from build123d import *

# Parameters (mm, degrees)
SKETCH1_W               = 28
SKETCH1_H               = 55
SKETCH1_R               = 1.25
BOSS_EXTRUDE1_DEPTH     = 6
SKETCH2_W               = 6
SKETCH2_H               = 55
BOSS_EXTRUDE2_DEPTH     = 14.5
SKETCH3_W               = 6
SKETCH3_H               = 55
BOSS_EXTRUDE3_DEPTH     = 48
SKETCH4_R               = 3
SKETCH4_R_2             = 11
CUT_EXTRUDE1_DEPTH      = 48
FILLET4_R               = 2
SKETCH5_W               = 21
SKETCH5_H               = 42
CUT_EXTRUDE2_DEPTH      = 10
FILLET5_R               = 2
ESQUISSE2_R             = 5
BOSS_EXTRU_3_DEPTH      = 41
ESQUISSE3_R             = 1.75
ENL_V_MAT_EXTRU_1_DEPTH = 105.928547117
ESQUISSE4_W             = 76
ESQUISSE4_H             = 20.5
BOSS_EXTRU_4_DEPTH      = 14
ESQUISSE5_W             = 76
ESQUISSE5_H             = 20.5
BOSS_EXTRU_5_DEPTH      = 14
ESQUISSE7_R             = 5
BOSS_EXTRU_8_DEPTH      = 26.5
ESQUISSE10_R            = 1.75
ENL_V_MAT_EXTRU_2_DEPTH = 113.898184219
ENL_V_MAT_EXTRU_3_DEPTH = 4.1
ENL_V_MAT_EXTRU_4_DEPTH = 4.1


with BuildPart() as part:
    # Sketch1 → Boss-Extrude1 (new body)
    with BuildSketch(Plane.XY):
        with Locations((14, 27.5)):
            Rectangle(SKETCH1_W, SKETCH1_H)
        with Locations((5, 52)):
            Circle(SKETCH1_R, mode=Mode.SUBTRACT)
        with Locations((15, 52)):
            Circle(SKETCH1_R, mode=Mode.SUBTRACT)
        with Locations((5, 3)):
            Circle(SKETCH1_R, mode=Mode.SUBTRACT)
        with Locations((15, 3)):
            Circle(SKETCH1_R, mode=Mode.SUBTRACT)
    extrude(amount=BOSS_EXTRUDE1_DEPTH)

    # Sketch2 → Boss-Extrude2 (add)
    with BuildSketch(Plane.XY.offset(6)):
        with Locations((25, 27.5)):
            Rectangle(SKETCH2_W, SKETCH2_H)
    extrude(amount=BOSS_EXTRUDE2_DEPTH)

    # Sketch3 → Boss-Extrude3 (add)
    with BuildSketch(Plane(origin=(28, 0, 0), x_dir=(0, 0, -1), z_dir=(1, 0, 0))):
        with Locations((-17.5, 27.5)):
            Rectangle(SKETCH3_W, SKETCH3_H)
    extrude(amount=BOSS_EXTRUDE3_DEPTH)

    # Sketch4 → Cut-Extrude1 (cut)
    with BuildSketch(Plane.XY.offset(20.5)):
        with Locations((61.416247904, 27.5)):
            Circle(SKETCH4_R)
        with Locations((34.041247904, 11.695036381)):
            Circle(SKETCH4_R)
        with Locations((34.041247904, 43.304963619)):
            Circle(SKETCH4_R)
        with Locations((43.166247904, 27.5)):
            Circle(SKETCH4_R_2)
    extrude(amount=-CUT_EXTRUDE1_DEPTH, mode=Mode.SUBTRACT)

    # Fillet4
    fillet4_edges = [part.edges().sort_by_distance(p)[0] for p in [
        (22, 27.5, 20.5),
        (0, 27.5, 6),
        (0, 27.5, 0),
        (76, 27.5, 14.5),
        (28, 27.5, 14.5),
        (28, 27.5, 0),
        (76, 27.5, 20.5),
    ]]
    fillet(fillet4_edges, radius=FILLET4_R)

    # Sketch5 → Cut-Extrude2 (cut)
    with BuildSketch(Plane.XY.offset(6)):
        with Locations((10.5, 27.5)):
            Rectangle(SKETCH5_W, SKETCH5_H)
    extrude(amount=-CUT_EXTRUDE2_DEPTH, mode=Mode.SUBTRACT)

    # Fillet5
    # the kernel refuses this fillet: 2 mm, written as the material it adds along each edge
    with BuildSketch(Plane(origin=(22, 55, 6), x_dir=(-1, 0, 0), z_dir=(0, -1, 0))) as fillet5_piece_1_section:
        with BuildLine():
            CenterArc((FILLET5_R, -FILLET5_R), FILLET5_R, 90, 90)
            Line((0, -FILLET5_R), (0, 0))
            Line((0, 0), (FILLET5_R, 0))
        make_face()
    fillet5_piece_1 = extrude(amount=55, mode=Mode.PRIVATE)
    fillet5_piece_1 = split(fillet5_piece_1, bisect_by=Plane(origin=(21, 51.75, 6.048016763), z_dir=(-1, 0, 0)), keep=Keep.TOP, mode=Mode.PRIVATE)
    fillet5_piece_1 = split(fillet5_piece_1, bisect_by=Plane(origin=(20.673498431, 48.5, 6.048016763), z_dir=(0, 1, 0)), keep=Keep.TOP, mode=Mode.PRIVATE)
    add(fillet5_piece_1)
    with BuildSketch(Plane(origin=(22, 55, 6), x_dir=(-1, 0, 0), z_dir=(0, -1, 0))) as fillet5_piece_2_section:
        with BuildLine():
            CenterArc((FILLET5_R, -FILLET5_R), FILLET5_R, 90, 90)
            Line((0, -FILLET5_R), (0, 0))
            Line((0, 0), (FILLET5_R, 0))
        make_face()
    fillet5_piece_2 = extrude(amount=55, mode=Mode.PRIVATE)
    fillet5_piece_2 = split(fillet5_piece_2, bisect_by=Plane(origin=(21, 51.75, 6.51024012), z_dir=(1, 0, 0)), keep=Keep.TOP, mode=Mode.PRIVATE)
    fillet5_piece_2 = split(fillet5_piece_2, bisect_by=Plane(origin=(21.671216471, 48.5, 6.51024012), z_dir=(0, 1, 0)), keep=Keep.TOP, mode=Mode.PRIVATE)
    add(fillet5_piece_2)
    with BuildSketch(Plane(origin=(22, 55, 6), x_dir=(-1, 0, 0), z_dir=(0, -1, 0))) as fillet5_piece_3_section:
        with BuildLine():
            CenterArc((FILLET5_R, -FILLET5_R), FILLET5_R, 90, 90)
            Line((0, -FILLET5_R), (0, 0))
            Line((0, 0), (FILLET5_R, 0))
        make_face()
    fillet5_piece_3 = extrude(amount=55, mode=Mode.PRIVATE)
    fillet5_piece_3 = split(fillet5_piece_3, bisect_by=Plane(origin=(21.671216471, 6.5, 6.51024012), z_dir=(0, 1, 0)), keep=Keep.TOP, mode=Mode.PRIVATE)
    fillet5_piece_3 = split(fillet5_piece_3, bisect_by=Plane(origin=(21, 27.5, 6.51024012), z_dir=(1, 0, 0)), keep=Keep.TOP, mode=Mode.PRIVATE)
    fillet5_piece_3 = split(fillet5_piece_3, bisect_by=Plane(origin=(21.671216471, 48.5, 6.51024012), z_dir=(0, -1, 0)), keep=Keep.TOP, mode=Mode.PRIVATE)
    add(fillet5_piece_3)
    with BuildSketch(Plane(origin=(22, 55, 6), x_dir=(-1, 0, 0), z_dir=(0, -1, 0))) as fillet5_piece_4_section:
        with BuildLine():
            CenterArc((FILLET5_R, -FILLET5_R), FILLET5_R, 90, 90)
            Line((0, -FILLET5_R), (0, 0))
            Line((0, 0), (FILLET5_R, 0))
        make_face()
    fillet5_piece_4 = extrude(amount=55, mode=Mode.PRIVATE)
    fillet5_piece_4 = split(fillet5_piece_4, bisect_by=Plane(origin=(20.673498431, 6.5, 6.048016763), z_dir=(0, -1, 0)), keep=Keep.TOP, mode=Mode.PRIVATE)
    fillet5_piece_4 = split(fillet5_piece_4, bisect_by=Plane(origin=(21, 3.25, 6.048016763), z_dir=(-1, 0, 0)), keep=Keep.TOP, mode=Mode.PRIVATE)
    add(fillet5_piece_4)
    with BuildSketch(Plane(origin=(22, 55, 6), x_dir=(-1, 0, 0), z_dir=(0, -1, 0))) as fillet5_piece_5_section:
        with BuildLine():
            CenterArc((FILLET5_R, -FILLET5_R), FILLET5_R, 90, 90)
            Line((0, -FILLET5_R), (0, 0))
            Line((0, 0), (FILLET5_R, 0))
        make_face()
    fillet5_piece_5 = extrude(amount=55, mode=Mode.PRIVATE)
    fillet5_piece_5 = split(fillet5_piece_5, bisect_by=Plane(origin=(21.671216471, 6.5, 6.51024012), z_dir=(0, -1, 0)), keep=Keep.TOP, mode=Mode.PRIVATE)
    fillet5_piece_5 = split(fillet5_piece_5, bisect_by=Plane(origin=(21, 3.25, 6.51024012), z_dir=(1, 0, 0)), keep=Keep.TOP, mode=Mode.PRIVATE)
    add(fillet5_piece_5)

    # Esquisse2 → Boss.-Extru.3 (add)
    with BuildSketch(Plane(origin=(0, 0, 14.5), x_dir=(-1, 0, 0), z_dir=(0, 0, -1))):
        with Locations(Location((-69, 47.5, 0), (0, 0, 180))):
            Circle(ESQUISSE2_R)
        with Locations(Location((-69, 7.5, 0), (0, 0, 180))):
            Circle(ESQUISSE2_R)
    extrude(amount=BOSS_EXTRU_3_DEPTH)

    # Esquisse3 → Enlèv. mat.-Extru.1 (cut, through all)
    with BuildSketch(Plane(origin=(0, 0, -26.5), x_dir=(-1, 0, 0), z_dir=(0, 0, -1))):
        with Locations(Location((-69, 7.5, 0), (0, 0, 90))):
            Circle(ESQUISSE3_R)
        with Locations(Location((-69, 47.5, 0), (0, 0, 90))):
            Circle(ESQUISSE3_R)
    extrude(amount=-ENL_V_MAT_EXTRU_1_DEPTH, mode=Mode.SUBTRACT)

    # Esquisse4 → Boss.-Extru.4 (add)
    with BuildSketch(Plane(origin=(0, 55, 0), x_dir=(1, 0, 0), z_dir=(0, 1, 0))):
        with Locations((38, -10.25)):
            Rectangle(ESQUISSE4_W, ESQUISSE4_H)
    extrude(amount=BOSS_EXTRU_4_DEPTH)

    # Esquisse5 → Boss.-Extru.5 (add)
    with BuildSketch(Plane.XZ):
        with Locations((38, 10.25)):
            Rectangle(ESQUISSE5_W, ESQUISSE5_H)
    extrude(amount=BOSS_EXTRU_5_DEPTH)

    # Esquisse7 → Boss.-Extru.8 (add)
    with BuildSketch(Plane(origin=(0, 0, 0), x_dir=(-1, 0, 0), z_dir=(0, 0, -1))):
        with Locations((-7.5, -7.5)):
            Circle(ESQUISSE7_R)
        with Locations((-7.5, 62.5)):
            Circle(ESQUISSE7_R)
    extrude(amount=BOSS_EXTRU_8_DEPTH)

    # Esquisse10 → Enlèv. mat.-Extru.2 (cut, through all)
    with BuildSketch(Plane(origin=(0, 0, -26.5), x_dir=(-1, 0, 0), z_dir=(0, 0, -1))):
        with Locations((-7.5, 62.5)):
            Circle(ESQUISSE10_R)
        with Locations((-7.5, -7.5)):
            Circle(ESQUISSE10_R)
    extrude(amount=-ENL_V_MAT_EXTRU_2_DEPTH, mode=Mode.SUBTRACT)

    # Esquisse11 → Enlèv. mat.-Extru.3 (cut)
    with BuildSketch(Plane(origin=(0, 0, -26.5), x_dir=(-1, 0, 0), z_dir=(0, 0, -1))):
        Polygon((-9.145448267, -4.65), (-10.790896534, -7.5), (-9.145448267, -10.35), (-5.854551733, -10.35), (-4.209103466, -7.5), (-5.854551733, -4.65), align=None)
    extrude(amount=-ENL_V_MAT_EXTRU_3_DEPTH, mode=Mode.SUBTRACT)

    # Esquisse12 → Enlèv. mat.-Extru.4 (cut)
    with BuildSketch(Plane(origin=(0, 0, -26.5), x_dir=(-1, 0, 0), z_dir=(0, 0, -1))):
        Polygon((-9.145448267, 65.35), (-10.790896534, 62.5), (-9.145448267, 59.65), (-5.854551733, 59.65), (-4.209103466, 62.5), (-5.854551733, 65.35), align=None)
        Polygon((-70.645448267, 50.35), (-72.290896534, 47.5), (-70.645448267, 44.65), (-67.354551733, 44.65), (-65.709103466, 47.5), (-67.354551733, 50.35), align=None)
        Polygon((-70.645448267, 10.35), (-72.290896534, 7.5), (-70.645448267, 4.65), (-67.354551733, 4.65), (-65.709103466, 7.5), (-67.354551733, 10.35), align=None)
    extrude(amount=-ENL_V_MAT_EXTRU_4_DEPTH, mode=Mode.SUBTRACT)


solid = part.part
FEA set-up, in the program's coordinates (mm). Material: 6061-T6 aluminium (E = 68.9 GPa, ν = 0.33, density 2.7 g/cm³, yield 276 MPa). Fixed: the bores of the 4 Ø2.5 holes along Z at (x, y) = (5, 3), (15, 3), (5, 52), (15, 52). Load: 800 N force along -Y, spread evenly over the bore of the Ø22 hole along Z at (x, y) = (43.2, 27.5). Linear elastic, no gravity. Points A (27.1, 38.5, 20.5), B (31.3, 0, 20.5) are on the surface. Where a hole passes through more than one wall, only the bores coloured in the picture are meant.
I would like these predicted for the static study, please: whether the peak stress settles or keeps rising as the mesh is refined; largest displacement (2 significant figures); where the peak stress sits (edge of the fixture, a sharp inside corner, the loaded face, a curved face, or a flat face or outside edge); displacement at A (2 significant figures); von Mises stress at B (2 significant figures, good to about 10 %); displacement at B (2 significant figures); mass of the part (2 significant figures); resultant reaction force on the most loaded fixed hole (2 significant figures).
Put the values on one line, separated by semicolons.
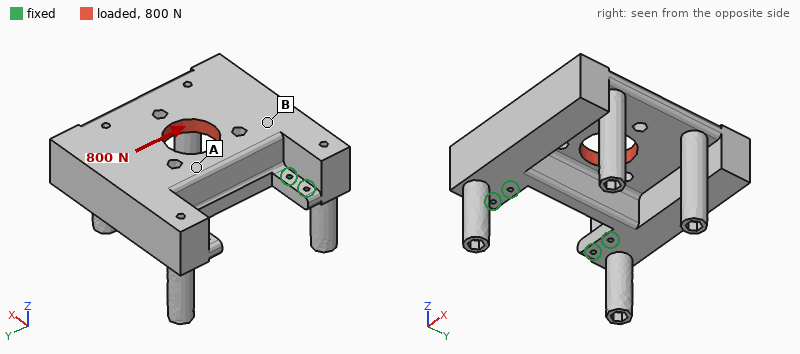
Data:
keeps rising; 13 µm; edge of the fixture; 5.4 µm; 3.5 MPa; 6.8 µm; 200 g; 710 N
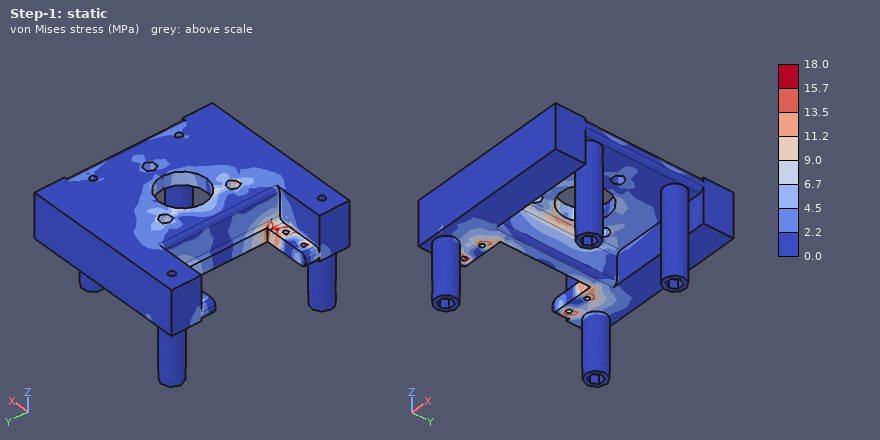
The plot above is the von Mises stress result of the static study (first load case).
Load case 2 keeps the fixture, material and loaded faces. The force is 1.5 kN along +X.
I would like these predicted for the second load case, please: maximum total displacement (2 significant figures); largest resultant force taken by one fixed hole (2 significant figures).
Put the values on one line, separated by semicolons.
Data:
63 µm; 870 N
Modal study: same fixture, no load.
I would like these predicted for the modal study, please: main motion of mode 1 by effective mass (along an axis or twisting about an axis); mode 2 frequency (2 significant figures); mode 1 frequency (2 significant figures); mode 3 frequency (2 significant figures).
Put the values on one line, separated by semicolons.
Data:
along Z; 1900 Hz; 1400 Hz; 2800 Hz
